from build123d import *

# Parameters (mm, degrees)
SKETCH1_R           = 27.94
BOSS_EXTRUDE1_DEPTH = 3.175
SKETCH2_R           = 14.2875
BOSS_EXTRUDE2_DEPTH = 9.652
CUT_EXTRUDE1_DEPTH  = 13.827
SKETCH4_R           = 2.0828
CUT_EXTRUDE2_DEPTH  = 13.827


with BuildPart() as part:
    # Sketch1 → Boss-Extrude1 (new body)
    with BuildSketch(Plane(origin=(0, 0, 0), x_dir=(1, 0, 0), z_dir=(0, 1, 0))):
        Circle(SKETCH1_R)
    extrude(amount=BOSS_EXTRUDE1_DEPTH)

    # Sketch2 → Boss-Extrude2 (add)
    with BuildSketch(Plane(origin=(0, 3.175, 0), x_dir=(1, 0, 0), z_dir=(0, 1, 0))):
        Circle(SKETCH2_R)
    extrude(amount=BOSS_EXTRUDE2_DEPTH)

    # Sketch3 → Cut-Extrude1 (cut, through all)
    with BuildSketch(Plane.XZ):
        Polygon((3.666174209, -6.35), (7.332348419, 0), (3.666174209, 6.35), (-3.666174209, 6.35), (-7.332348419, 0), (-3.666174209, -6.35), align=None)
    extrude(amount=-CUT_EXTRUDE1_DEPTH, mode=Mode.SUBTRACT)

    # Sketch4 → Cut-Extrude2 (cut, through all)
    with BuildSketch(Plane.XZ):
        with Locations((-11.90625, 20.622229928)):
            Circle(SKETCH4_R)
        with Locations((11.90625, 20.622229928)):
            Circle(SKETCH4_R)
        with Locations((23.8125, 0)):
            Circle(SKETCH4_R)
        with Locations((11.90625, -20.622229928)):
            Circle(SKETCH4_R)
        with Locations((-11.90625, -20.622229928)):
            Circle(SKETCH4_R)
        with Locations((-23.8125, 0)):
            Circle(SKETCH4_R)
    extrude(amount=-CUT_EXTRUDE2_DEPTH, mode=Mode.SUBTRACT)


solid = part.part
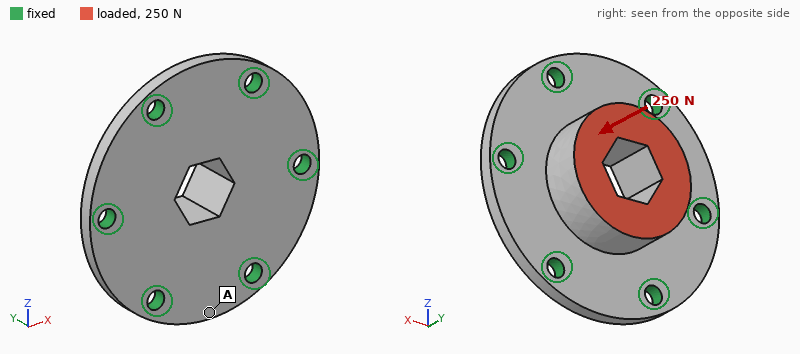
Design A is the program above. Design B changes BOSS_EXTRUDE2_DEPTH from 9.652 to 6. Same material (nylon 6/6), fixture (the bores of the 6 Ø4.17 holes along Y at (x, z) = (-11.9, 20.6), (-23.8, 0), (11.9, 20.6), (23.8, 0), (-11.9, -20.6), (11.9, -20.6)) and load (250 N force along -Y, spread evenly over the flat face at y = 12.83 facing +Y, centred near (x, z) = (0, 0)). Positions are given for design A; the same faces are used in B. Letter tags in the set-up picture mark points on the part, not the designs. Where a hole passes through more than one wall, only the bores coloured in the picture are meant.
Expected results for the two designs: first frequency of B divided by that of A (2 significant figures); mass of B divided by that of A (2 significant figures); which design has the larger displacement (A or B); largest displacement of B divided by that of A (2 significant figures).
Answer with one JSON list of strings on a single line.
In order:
["1.1", "0.85", "B", "1.1"]
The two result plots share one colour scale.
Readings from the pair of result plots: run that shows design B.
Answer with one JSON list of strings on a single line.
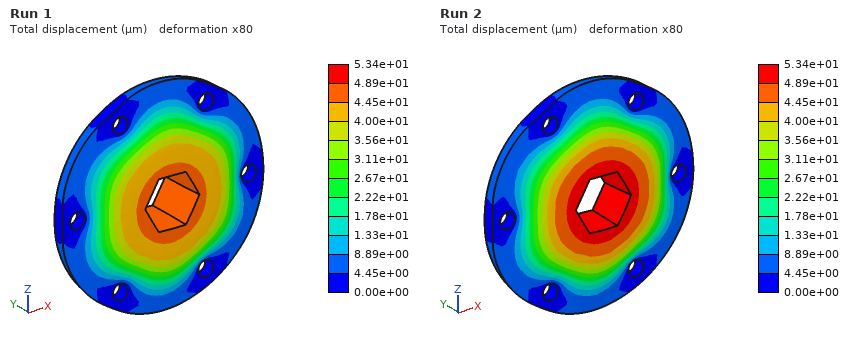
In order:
["Run 2"]
